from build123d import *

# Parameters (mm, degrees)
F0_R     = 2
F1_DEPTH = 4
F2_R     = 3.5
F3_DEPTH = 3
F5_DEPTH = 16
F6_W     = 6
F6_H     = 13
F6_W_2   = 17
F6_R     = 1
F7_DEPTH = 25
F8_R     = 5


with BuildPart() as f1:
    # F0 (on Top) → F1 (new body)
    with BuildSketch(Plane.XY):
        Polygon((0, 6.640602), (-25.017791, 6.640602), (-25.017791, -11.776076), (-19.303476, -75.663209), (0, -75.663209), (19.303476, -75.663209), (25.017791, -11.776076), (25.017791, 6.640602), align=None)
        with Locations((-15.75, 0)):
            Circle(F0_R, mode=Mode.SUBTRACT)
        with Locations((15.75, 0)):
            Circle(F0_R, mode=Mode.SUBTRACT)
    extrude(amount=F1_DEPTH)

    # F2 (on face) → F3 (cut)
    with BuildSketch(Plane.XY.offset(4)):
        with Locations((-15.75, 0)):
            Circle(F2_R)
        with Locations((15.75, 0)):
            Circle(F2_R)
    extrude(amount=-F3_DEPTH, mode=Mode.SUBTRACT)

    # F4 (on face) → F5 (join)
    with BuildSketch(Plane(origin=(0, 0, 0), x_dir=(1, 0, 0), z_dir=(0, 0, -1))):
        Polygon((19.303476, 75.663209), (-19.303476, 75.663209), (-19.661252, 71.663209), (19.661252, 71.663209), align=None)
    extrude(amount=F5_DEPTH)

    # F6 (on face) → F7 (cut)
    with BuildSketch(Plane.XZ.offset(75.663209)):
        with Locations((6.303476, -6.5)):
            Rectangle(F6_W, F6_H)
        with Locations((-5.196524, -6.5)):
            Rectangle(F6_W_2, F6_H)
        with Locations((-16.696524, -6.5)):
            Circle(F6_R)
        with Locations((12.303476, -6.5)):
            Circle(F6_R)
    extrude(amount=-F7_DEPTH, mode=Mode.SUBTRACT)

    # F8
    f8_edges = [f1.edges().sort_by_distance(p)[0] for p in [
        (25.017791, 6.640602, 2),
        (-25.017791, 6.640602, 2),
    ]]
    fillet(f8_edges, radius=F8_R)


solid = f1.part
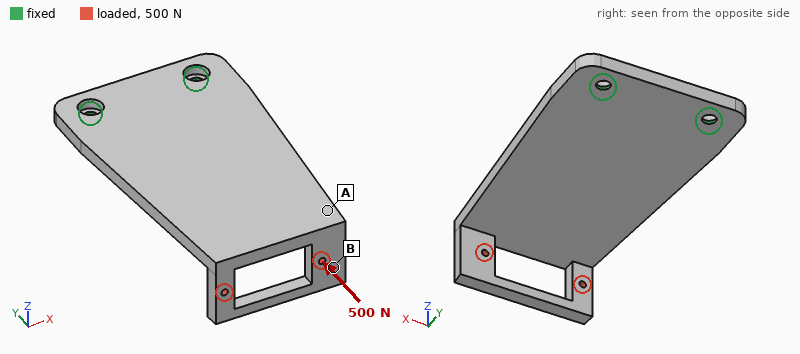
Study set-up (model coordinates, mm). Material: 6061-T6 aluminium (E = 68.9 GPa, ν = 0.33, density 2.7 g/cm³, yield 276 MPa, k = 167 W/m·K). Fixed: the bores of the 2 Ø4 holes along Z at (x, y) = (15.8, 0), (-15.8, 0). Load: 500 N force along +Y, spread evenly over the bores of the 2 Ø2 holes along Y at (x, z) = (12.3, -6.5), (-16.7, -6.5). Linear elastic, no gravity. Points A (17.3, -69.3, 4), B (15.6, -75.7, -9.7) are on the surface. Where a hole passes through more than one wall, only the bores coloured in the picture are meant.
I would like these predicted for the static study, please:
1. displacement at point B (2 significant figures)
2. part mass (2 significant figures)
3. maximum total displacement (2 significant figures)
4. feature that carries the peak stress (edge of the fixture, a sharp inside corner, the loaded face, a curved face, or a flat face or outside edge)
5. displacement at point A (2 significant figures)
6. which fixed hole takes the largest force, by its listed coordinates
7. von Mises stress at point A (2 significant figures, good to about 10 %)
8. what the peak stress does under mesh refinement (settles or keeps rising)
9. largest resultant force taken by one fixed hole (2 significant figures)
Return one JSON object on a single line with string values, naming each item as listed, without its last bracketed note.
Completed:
{"displacement at point B": "1.1 mm", "part mass": "43 g", "maximum total displacement": "1.2 mm", "feature that carries the peak stress": "edge of the fixture", "displacement at point A": "0.91 mm", "which fixed hole takes the largest force, by its listed coordinates": "(-15.8, 0)", "von Mises stress at point A": "46 MPa", "what the peak stress does under mesh refinement": "keeps rising", "largest resultant force taken by one fixed hole": "300 N"}
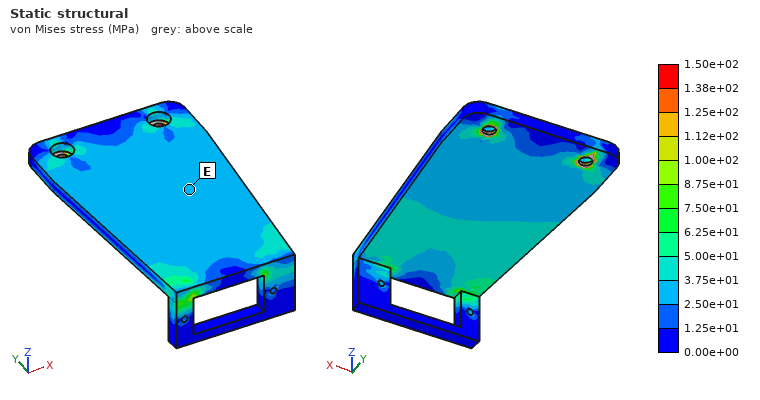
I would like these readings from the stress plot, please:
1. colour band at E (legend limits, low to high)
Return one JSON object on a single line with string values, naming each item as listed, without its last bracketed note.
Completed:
{"colour band at E": "2.50e+01 to 3.75e+01 MPa"}
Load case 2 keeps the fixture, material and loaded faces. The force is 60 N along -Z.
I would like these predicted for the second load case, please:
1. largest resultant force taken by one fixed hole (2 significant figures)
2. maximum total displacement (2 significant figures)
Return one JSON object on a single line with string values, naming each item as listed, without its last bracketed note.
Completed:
{"largest resultant force taken by one fixed hole": "80 N", "maximum total displacement": "0.98 mm"}
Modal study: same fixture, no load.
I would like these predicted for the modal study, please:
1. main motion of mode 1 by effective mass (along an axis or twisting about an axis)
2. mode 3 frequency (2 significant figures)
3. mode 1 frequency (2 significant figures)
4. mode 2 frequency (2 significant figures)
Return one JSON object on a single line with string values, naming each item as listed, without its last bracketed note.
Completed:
{"main motion of mode 1 by effective mass": "along Z", "mode 3 frequency": "2300 Hz", "mode 1 frequency": "350 Hz", "mode 2 frequency": "1700 Hz"}
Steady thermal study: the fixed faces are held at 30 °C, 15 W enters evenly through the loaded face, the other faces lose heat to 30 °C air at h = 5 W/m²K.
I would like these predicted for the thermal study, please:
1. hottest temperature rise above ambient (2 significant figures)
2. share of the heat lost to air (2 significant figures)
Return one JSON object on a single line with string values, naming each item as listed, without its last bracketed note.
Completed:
{"hottest temperature rise above ambient": "58 K", "share of the heat lost to air": "7.5 %"}
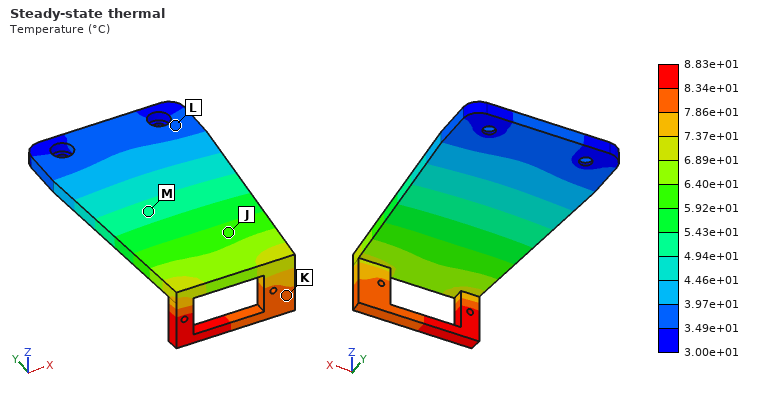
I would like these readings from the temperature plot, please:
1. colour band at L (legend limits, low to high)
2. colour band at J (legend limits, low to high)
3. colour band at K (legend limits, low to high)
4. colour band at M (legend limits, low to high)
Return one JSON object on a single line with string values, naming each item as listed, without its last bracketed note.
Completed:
{"colour band at L": "3.49e+01 to 3.97e+01 °C", "colour band at J": "5.92e+01 to 6.40e+01 °C", "colour band at K": "7.86e+01 to 8.34e+01 °C", "colour band at M": "4.94e+01 to 5.43e+01 °C"}
